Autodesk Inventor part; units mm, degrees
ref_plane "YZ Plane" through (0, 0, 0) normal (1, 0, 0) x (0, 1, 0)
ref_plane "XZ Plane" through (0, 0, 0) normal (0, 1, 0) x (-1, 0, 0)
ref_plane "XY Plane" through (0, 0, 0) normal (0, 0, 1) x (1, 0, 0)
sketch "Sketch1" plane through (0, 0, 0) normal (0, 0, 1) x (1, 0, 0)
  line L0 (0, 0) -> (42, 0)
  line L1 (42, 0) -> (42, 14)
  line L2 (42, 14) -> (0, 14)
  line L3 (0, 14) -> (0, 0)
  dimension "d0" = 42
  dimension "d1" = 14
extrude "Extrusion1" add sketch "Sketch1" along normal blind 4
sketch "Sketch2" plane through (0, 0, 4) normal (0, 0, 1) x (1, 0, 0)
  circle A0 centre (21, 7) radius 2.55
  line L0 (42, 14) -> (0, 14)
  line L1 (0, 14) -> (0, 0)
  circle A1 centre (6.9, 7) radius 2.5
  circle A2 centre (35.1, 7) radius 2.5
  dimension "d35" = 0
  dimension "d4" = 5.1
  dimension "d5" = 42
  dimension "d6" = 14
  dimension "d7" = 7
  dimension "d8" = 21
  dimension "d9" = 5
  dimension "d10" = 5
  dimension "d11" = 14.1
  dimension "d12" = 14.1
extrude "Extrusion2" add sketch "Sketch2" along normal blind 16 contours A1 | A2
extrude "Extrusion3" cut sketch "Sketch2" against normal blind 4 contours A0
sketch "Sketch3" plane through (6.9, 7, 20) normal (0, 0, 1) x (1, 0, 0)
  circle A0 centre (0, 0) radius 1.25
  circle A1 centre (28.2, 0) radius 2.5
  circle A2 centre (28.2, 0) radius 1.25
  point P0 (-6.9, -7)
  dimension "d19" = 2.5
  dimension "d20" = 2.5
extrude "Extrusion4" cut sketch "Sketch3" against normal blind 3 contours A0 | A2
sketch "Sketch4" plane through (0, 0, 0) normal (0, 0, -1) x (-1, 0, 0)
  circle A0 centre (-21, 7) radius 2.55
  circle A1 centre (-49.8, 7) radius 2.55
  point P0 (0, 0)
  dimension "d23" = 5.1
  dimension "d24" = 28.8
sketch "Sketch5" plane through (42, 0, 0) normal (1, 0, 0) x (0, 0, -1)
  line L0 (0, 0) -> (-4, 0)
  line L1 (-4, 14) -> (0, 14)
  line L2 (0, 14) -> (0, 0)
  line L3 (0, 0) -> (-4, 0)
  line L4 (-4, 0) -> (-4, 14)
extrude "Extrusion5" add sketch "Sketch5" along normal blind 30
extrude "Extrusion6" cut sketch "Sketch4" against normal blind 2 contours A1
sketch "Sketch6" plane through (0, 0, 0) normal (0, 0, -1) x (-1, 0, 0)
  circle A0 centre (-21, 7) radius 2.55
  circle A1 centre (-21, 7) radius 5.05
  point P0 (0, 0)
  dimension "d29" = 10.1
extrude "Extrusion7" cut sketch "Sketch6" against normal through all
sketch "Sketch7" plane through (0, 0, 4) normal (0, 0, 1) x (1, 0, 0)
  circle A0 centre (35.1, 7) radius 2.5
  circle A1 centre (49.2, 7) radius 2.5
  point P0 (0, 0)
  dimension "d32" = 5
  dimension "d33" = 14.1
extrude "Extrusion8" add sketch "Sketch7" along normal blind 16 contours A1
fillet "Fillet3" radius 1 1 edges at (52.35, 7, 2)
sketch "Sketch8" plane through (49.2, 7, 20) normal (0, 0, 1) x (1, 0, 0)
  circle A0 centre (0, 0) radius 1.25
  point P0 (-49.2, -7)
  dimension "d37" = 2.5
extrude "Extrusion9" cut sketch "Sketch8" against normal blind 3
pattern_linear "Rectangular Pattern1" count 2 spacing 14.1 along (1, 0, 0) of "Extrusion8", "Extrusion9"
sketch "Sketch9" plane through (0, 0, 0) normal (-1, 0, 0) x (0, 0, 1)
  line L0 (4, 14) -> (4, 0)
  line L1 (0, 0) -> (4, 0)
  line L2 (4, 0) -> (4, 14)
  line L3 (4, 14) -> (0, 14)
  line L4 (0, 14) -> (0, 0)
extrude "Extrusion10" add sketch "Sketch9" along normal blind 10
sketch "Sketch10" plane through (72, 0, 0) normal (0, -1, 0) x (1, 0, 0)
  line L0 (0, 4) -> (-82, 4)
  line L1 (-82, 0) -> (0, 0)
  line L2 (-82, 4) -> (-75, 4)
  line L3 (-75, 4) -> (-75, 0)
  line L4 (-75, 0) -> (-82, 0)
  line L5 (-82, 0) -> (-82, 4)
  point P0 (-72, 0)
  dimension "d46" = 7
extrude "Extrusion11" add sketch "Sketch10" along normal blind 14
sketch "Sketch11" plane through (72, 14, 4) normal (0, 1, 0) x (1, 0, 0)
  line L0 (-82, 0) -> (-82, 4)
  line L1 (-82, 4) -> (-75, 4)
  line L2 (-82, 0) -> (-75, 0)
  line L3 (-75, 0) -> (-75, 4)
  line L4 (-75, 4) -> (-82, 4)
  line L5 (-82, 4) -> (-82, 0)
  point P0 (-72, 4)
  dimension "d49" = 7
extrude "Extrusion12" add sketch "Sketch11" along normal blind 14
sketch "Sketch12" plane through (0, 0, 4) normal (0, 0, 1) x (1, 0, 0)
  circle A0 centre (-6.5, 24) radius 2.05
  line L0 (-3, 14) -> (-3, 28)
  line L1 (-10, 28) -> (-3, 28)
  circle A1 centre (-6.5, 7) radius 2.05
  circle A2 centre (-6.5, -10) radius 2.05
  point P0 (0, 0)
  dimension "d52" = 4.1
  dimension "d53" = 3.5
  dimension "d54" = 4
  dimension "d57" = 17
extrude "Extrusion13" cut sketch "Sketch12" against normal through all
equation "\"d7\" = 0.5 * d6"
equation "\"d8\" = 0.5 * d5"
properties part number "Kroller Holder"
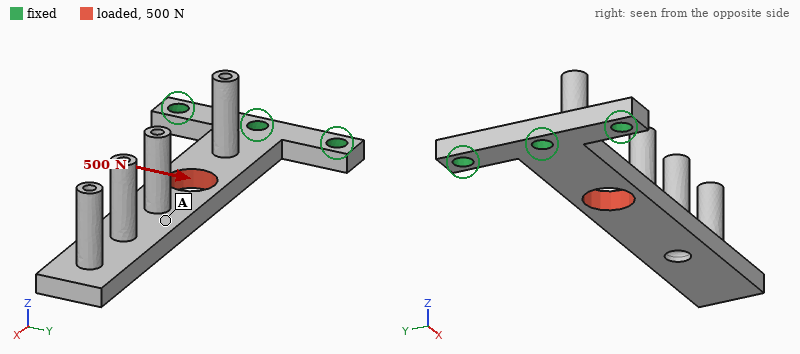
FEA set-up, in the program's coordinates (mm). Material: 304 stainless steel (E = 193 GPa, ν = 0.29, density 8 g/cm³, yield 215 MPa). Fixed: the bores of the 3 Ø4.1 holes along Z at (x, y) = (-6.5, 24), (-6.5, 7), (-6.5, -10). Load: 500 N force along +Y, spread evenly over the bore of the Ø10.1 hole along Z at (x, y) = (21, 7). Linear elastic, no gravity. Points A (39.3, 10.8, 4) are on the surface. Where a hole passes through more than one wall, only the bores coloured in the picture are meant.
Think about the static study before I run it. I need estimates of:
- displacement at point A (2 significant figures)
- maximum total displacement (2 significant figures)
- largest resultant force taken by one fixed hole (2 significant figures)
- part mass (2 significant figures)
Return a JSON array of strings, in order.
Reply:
["0.061 mm", "0.11 mm", "370 N", "48 g"]
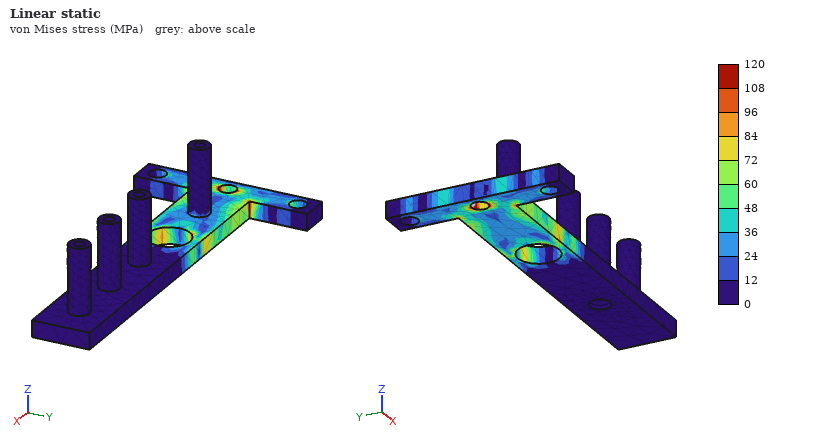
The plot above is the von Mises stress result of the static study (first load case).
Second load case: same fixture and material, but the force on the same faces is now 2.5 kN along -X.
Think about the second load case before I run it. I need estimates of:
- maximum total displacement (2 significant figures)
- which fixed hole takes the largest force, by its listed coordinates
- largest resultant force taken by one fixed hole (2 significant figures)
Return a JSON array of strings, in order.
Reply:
["11 µm", "(-6.5, 7)", "2.2 kN"]
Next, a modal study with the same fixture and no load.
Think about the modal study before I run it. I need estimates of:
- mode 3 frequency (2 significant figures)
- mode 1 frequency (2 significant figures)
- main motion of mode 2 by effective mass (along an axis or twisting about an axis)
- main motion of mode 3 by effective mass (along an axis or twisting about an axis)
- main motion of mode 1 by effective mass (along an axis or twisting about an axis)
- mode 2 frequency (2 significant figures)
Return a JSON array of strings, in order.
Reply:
["2700 Hz", "400 Hz", "along Y", "twisting about X", "along Z", "1300 Hz"]
